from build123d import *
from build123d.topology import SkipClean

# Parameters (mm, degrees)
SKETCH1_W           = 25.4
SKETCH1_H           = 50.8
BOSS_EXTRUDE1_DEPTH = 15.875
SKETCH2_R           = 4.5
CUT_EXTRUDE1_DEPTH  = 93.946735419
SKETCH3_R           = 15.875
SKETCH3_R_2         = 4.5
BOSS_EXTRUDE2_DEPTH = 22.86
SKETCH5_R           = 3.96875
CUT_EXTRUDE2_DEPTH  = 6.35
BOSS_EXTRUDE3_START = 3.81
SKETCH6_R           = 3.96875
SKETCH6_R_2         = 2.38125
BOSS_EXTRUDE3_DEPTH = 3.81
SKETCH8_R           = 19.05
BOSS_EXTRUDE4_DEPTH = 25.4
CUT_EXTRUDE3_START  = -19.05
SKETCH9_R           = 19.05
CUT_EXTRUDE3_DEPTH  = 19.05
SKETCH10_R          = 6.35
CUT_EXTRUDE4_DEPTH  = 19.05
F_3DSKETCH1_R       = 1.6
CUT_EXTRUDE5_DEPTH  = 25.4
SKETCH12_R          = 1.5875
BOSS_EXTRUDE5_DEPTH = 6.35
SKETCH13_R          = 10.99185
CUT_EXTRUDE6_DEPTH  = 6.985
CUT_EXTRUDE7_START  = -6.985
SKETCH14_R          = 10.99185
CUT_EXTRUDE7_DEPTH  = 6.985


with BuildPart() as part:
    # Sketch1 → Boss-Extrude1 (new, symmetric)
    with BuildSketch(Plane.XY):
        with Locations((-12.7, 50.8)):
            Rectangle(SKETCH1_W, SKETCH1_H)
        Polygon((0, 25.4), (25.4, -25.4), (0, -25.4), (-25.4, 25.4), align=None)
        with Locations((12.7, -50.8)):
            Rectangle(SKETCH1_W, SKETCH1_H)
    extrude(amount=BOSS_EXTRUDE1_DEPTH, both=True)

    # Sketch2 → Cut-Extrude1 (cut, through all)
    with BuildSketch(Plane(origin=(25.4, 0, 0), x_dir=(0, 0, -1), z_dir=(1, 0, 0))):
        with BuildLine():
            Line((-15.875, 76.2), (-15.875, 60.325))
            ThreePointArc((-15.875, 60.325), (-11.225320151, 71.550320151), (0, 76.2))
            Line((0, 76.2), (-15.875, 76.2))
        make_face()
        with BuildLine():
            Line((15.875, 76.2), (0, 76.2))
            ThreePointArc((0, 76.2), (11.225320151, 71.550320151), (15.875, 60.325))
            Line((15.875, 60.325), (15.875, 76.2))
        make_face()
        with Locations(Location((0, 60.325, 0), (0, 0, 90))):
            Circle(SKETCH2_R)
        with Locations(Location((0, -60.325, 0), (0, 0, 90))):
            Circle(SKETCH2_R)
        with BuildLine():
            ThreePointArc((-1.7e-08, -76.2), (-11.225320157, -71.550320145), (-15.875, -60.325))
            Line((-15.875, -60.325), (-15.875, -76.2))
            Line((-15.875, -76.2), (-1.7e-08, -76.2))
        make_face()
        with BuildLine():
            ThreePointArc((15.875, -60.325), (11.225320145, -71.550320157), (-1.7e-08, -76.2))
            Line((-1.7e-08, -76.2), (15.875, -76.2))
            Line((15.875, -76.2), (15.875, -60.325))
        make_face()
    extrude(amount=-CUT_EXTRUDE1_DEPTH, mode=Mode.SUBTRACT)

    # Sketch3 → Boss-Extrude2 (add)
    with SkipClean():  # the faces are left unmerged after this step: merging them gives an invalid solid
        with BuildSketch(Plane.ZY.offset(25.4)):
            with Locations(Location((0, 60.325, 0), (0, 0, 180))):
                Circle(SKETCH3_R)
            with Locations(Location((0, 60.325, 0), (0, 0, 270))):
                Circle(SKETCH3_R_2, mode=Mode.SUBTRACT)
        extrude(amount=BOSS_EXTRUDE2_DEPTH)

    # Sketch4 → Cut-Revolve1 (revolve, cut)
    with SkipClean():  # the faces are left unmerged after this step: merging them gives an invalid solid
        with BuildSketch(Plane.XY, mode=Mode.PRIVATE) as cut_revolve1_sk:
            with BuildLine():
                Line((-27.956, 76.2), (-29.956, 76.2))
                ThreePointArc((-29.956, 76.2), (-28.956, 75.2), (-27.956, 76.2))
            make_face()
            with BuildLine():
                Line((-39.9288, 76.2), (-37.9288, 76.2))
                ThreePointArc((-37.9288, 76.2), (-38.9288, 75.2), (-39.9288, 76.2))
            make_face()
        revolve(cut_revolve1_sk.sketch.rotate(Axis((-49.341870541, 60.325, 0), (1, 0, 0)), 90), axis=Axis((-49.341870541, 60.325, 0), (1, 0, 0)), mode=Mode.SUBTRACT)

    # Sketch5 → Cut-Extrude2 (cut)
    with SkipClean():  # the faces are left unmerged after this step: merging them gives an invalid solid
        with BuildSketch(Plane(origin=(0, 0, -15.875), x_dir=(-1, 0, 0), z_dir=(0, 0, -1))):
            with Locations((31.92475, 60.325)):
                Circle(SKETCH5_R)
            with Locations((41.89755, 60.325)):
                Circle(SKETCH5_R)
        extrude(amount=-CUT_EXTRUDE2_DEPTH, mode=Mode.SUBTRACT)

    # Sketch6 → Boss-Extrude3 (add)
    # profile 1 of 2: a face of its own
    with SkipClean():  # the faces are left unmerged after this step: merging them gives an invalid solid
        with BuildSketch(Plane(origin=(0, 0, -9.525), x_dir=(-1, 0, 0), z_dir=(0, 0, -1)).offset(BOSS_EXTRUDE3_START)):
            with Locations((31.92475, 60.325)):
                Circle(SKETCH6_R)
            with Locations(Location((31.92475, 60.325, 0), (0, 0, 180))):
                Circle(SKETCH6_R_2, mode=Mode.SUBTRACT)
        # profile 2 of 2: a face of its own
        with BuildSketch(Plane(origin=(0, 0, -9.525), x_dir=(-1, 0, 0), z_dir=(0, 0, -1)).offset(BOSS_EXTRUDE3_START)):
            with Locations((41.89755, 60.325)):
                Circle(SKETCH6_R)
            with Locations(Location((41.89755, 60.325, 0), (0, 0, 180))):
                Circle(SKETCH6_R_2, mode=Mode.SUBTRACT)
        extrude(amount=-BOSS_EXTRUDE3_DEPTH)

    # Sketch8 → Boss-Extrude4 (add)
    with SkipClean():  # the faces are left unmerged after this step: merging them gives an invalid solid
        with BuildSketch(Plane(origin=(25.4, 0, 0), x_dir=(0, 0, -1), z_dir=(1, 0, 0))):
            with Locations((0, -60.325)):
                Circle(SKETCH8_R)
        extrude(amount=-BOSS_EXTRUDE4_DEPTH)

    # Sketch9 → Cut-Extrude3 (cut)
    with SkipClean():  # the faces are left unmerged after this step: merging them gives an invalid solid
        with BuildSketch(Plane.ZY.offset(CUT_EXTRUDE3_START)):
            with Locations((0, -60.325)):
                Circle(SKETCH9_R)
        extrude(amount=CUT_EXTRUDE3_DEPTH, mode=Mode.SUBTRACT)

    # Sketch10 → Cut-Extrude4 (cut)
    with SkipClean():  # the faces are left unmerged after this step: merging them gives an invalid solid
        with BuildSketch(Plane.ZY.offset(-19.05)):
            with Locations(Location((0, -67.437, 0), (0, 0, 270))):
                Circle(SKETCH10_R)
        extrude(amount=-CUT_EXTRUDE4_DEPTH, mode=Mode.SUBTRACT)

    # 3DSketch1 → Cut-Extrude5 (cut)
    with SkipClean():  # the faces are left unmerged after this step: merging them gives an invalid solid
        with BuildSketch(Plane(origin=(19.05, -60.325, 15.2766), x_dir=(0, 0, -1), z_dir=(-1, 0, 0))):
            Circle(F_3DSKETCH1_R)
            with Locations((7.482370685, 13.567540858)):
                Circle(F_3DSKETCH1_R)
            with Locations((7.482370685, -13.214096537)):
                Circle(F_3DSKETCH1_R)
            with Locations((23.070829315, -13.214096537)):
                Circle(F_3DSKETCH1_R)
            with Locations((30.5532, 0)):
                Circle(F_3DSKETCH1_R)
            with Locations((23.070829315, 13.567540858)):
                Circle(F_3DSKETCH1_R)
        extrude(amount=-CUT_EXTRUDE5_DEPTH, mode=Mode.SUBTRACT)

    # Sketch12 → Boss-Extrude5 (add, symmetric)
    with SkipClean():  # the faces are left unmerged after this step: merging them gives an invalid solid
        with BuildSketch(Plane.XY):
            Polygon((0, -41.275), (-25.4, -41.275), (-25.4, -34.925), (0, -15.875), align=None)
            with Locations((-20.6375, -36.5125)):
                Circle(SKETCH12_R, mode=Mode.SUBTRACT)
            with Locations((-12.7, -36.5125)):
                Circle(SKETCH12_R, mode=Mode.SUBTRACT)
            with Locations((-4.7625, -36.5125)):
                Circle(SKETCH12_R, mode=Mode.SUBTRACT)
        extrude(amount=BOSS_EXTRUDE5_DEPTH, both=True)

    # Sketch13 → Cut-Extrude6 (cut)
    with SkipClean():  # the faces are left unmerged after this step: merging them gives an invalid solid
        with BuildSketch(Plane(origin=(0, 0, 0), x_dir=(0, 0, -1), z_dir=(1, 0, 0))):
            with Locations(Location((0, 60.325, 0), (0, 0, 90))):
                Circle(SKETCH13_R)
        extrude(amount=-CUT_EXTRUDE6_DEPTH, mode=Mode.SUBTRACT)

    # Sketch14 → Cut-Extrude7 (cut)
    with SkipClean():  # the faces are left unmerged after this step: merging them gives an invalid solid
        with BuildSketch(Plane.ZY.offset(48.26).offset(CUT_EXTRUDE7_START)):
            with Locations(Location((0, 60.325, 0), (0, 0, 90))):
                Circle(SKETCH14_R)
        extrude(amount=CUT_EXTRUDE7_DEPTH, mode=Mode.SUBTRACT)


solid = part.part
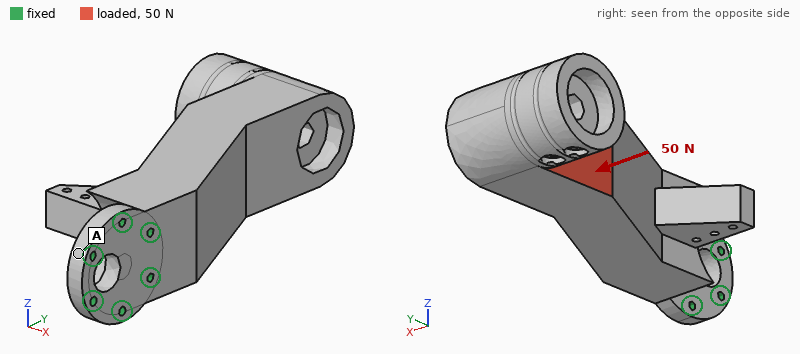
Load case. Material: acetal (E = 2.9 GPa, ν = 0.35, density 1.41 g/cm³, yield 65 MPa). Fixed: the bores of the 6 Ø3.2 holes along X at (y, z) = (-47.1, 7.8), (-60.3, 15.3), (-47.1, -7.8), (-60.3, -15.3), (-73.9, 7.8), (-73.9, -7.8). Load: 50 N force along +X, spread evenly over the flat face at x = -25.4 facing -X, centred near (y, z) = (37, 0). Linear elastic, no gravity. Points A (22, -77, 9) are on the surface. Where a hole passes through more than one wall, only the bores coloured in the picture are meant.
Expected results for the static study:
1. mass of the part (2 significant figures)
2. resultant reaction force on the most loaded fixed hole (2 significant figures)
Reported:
160 g
90 N
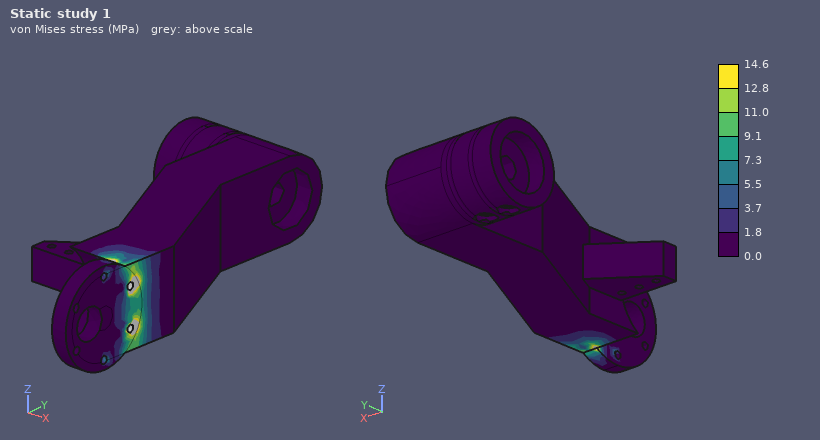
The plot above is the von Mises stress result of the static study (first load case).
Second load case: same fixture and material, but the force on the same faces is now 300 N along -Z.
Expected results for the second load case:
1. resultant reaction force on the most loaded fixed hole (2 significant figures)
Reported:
1.1 kN
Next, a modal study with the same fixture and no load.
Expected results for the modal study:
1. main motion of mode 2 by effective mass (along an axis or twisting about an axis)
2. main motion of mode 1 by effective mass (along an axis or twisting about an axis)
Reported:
along Z
along X
